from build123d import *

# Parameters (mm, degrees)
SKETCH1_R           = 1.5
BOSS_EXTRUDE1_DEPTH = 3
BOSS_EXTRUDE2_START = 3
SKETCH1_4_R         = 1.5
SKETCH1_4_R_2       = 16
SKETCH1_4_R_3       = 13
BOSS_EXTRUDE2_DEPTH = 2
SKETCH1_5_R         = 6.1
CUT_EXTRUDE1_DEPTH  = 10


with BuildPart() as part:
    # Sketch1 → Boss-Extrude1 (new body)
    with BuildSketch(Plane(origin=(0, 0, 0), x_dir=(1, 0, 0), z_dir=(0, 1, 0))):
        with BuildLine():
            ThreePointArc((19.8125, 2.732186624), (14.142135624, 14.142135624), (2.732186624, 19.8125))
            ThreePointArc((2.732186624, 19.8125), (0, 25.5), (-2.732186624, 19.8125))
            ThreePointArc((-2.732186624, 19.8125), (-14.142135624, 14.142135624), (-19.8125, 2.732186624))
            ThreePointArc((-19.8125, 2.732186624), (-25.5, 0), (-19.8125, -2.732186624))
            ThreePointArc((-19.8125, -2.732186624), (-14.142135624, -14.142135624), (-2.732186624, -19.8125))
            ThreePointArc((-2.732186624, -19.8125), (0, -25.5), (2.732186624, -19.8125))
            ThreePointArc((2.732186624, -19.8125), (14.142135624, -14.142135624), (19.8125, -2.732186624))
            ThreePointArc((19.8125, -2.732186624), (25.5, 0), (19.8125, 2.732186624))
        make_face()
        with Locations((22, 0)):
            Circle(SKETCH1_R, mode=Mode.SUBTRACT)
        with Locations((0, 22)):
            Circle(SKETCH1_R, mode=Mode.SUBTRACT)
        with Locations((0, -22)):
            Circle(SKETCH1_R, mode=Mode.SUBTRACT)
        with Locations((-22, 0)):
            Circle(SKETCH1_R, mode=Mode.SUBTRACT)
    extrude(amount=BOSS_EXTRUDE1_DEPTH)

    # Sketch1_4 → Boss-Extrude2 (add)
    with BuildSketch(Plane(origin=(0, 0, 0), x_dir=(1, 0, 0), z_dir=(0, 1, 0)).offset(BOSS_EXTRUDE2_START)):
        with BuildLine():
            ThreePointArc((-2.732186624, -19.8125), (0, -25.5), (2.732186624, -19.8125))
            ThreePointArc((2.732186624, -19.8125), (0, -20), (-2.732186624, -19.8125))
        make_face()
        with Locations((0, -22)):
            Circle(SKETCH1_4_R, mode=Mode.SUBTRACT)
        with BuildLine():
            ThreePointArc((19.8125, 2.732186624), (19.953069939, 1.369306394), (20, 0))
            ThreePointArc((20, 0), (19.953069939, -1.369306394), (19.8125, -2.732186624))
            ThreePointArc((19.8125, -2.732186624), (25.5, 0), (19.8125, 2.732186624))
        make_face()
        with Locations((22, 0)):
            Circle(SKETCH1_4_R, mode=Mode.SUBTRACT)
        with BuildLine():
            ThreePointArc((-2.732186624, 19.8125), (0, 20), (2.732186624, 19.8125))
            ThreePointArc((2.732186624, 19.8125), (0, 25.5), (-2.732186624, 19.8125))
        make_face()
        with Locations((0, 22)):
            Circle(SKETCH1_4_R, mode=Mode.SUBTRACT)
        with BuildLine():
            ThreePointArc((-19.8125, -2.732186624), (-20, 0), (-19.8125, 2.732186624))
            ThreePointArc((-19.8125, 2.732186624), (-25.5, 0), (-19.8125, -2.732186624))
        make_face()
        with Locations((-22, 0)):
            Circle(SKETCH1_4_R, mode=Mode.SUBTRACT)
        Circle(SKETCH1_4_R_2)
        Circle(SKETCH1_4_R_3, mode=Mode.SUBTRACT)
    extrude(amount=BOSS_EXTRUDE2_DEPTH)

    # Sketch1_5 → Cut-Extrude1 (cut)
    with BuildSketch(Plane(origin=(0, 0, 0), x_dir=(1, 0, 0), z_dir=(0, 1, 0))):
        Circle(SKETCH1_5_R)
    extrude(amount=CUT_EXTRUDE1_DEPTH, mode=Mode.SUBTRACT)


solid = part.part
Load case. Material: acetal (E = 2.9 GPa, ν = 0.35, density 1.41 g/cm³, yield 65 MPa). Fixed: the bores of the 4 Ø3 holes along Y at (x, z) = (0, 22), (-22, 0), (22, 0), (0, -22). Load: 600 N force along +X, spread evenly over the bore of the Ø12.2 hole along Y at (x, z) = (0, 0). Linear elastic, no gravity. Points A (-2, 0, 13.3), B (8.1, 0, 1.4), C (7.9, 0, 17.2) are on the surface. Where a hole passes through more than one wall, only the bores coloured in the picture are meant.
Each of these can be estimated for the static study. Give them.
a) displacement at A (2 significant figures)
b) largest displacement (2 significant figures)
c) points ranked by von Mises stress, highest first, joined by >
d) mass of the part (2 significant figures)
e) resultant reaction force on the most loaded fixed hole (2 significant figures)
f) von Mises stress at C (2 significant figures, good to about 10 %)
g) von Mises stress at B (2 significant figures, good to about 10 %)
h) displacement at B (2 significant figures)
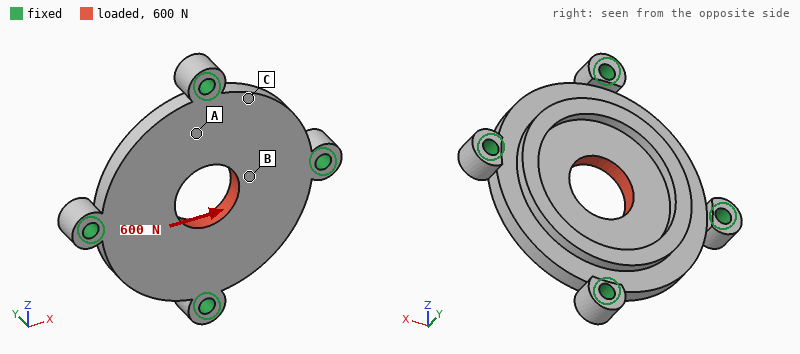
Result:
27 µm
49 µm
B > C > A
6.3 g
220 N
3.0 MPa
6.8 MPa
37 µm
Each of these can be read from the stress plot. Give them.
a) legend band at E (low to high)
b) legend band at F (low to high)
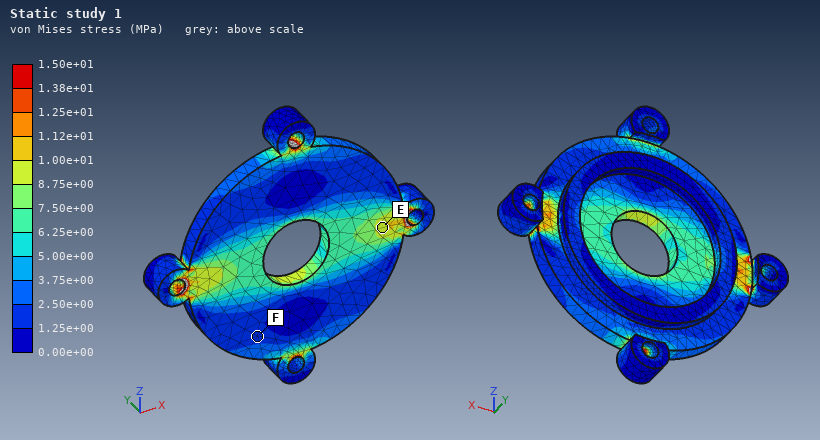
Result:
8.75e+00 to 1.00e+01 MPa
1.25e+00 to 2.50e+00 MPa
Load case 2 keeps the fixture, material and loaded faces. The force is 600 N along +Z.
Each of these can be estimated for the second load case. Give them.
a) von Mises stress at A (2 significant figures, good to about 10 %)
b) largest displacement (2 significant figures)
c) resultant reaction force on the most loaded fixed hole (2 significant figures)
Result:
8.1 MPa
49 µm
220 N
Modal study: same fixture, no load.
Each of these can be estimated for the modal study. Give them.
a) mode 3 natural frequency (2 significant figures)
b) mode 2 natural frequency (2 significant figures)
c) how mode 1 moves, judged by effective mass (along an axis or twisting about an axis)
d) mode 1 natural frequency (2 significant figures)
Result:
4900 Hz
4700 Hz
along Y
3500 Hz
